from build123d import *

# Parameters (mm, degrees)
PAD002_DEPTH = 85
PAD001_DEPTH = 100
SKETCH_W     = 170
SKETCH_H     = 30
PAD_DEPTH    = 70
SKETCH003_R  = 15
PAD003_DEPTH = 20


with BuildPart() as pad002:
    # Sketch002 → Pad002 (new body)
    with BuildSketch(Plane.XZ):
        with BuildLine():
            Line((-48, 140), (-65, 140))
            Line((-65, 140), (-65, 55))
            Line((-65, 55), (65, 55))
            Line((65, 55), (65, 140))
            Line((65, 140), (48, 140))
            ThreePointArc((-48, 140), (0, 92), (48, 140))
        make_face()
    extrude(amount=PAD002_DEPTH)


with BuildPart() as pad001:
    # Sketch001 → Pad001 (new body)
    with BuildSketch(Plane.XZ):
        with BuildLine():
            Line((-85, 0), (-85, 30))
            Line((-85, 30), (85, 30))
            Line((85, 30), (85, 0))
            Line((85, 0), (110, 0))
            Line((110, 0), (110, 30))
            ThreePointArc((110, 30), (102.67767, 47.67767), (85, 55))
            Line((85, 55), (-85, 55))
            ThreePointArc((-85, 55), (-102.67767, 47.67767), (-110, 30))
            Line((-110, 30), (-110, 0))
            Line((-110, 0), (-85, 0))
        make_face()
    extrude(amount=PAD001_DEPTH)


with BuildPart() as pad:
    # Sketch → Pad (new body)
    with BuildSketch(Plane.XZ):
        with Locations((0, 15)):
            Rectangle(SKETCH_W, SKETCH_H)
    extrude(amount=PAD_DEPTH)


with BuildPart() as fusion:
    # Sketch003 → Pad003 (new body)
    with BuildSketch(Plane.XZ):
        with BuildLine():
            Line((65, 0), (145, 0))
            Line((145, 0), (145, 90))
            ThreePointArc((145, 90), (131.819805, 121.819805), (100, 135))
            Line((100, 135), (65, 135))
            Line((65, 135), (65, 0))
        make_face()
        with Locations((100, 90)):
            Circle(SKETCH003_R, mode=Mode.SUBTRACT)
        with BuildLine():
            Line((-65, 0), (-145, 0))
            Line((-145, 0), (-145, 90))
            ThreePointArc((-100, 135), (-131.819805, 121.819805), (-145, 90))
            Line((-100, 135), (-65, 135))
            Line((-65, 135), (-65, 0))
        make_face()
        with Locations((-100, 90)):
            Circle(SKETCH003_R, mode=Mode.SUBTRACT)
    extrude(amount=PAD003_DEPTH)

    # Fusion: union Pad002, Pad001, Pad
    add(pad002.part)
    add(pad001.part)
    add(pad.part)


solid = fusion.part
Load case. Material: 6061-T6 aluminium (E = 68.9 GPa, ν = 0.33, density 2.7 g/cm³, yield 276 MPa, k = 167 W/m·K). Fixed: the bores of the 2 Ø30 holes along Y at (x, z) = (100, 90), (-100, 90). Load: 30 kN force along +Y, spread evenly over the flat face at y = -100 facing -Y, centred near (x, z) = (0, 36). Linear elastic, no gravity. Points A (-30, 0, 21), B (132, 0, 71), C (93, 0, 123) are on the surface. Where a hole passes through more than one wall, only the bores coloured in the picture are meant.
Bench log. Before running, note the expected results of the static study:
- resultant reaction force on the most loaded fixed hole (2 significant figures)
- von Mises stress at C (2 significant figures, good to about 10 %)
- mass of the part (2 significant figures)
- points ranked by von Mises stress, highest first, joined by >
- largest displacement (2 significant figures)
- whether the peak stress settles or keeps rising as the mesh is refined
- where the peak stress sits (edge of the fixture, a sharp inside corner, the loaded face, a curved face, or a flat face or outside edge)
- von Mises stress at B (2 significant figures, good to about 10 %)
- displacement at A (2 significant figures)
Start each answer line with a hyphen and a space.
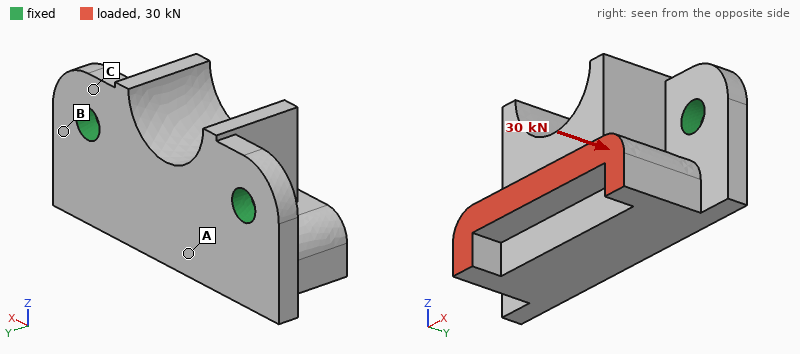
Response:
- 15 kN
- 24 MPa
- 5.3 kg
- B > C > A
- 0.24 mm
- keeps rising
- edge of the fixture
- 32 MPa
- 0.13 mm
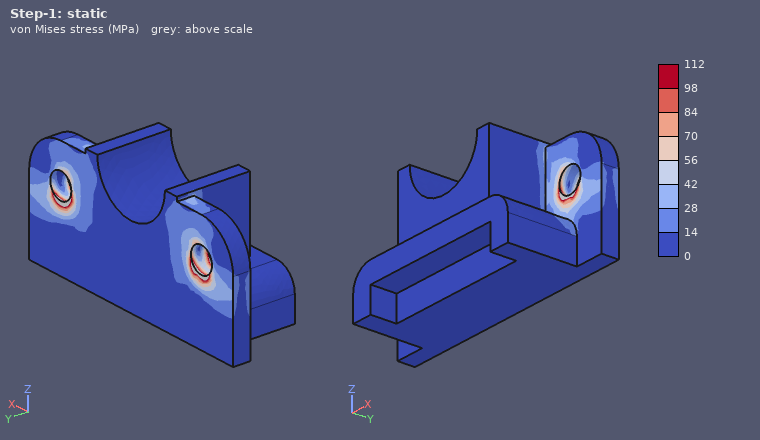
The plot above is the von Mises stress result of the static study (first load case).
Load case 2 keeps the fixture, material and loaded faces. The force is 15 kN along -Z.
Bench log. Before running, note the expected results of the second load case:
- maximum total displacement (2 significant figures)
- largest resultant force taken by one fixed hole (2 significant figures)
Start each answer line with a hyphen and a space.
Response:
- 0.25 mm
- 8.3 kN
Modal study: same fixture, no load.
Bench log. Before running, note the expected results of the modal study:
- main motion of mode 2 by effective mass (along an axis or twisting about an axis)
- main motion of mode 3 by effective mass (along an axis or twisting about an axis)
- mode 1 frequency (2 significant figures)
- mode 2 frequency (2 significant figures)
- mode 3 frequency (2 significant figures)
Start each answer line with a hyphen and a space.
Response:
- along X
- along Y
- 990 Hz
- 2800 Hz
- 2900 Hz
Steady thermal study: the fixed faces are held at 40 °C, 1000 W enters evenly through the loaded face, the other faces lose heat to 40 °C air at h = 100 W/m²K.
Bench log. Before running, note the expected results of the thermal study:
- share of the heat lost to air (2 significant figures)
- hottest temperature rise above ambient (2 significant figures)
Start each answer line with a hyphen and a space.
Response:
- 44 %
- 79 K
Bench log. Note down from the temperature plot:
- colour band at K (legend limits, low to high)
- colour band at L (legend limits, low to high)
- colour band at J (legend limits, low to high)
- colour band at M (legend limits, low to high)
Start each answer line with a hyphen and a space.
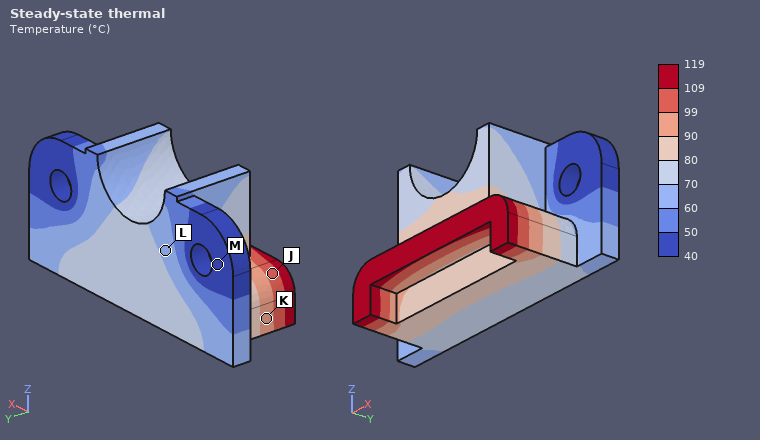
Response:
- 90 to 99 °C
- 60 to 70 °C
- 99 to 109 °C
- 40 to 50 °C
